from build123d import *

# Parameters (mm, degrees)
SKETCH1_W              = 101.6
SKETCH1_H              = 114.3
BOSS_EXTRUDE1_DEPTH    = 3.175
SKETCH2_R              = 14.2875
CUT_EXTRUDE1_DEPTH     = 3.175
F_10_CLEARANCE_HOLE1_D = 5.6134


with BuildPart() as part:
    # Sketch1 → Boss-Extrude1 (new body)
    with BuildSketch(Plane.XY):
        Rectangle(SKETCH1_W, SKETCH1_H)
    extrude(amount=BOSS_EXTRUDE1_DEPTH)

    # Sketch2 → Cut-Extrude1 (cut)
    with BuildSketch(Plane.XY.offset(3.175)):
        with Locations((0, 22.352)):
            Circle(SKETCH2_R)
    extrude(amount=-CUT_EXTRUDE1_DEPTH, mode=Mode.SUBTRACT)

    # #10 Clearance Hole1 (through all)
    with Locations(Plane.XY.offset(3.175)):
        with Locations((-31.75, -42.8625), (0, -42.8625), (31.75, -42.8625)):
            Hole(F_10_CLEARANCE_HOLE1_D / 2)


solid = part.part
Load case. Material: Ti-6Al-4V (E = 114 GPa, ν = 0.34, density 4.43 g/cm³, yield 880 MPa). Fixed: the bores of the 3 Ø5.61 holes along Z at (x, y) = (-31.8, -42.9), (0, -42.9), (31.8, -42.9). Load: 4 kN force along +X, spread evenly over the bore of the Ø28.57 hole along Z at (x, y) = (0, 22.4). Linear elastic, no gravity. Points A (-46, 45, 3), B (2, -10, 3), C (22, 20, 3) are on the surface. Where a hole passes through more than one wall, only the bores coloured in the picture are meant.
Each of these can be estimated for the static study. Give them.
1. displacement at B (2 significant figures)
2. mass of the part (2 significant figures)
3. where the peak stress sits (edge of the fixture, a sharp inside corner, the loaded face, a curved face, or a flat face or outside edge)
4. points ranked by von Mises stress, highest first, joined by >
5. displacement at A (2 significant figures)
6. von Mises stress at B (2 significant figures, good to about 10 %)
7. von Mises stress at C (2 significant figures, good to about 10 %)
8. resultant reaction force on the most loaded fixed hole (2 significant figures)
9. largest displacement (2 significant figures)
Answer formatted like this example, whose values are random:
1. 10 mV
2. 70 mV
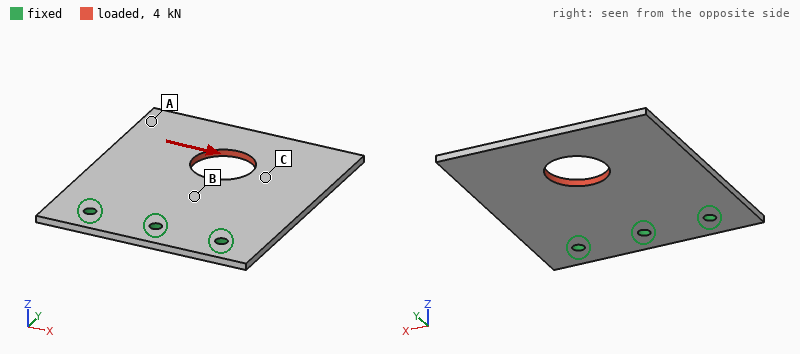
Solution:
1. 21 µm
2. 150 g
3. edge of the fixture
4. B > C > A
5. 67 µm
6. 42 MPa
7. 27 MPa
8. 4.1 kN
9. 75 µm
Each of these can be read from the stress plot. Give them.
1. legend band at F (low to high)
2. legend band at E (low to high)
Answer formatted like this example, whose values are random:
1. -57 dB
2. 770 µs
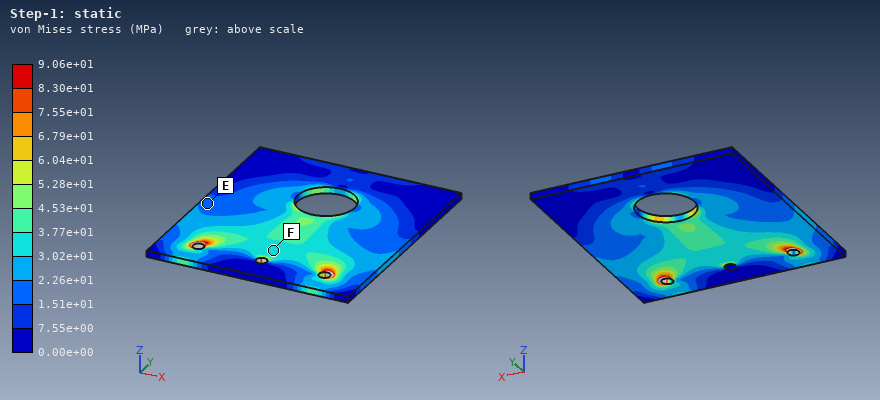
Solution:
1. 3.02e+01 to 3.77e+01 MPa
2. 1.51e+01 to 2.26e+01 MPa
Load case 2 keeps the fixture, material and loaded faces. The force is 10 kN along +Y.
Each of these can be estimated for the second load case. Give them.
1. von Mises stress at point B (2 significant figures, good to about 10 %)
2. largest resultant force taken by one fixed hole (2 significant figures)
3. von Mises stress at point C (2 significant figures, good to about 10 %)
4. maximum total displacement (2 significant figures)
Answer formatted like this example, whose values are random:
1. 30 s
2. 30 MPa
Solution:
1. 41 MPa
2. 3.5 kN
3. 44 MPa
4. 41 µm
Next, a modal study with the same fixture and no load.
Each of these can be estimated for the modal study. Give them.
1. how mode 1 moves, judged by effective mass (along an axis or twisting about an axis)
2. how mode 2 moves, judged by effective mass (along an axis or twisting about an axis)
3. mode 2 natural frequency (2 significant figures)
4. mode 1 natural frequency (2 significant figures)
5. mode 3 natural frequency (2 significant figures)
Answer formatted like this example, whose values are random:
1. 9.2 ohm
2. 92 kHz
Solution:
1. along Z
2. twisting about Y
3. 600 Hz
4. 270 Hz
5. 1500 Hz
